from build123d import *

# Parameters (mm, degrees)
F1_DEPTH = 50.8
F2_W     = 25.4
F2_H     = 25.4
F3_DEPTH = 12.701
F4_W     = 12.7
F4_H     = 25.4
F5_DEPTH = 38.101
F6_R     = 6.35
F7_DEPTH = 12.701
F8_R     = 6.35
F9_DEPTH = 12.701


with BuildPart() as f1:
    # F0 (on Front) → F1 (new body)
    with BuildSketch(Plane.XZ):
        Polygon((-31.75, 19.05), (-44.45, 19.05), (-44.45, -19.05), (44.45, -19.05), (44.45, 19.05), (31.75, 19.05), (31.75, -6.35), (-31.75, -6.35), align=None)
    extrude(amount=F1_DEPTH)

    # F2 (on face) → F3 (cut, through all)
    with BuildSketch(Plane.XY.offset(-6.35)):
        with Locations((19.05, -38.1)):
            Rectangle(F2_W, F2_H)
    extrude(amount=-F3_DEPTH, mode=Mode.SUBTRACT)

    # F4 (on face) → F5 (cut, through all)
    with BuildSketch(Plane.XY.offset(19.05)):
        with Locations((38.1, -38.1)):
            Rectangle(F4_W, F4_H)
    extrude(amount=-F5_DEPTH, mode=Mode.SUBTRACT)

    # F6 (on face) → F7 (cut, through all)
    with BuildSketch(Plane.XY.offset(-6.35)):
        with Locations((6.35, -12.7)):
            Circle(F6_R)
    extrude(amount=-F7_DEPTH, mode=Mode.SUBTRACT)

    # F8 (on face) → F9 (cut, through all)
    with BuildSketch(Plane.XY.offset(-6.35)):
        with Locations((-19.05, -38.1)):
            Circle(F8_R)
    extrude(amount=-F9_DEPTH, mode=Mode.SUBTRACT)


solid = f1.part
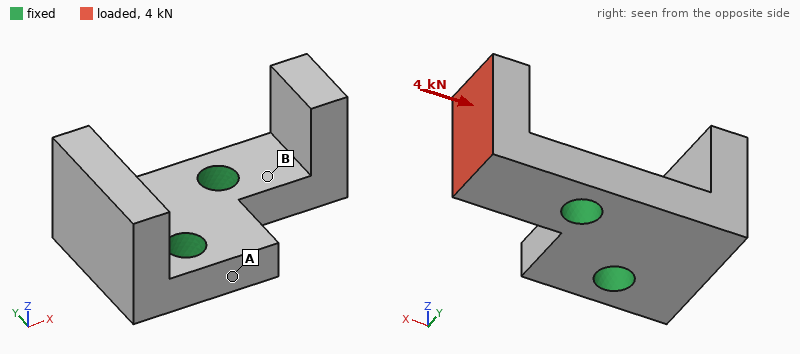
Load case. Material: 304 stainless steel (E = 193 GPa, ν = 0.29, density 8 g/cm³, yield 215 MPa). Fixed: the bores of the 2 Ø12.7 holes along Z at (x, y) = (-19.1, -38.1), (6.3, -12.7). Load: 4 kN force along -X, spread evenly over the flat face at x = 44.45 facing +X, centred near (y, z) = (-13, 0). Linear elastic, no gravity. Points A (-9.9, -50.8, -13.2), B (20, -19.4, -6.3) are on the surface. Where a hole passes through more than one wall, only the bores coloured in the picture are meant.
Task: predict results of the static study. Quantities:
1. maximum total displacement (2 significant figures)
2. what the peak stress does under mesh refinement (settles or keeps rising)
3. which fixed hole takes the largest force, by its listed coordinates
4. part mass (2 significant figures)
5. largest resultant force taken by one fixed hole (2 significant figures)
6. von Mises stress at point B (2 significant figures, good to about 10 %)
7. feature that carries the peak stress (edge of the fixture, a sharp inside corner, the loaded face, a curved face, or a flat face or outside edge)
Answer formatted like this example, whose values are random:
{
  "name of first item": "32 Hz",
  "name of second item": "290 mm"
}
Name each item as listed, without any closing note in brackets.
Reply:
{
  "maximum total displacement": "73 µm",
  "what the peak stress does under mesh refinement": "keeps rising",
  "which fixed hole takes the largest force, by its listed coordinates": "(6.3, -12.7)",
  "part mass": "530 g",
  "largest resultant force taken by one fixed hole": "3.9 kN",
  "von Mises stress at point B": "84 MPa",
  "feature that carries the peak stress": "edge of the fixture"
}
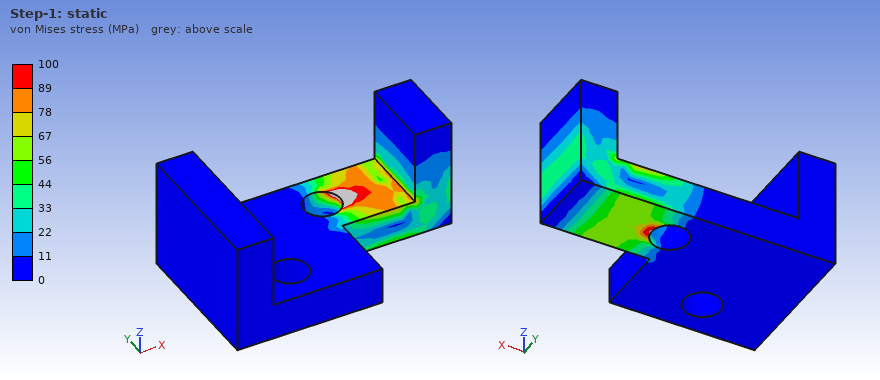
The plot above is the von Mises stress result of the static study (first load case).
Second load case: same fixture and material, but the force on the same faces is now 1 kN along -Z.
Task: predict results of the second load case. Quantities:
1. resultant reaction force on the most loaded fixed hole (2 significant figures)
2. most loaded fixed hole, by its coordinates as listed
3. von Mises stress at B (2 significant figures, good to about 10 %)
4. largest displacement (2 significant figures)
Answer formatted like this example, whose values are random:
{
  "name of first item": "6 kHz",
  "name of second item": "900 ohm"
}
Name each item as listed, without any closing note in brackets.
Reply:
{
  "resultant reaction force on the most loaded fixed hole": "1.1 kN",
  "most loaded fixed hole, by its coordinates as listed": "(6.3, -12.7)",
  "von Mises stress at B": "34 MPa",
  "largest displacement": "29 µm"
}
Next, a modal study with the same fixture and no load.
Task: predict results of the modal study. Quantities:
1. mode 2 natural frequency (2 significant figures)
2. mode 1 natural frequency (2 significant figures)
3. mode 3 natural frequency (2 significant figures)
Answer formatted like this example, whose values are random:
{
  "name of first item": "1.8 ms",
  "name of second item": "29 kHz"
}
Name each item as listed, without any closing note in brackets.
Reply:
{
  "mode 2 natural frequency": "4500 Hz",
  "mode 1 natural frequency": "3700 Hz",
  "mode 3 natural frequency": "4700 Hz"
}
